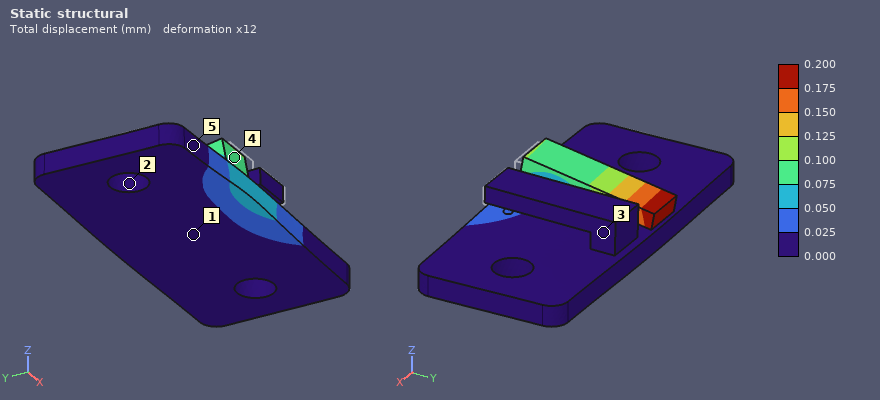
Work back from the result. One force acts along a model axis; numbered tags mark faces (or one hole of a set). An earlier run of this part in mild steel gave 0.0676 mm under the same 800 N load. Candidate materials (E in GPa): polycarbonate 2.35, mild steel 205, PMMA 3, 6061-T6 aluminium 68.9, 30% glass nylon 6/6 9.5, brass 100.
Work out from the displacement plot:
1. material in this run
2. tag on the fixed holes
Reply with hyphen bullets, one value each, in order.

- 6061-T6 aluminium
- 2
